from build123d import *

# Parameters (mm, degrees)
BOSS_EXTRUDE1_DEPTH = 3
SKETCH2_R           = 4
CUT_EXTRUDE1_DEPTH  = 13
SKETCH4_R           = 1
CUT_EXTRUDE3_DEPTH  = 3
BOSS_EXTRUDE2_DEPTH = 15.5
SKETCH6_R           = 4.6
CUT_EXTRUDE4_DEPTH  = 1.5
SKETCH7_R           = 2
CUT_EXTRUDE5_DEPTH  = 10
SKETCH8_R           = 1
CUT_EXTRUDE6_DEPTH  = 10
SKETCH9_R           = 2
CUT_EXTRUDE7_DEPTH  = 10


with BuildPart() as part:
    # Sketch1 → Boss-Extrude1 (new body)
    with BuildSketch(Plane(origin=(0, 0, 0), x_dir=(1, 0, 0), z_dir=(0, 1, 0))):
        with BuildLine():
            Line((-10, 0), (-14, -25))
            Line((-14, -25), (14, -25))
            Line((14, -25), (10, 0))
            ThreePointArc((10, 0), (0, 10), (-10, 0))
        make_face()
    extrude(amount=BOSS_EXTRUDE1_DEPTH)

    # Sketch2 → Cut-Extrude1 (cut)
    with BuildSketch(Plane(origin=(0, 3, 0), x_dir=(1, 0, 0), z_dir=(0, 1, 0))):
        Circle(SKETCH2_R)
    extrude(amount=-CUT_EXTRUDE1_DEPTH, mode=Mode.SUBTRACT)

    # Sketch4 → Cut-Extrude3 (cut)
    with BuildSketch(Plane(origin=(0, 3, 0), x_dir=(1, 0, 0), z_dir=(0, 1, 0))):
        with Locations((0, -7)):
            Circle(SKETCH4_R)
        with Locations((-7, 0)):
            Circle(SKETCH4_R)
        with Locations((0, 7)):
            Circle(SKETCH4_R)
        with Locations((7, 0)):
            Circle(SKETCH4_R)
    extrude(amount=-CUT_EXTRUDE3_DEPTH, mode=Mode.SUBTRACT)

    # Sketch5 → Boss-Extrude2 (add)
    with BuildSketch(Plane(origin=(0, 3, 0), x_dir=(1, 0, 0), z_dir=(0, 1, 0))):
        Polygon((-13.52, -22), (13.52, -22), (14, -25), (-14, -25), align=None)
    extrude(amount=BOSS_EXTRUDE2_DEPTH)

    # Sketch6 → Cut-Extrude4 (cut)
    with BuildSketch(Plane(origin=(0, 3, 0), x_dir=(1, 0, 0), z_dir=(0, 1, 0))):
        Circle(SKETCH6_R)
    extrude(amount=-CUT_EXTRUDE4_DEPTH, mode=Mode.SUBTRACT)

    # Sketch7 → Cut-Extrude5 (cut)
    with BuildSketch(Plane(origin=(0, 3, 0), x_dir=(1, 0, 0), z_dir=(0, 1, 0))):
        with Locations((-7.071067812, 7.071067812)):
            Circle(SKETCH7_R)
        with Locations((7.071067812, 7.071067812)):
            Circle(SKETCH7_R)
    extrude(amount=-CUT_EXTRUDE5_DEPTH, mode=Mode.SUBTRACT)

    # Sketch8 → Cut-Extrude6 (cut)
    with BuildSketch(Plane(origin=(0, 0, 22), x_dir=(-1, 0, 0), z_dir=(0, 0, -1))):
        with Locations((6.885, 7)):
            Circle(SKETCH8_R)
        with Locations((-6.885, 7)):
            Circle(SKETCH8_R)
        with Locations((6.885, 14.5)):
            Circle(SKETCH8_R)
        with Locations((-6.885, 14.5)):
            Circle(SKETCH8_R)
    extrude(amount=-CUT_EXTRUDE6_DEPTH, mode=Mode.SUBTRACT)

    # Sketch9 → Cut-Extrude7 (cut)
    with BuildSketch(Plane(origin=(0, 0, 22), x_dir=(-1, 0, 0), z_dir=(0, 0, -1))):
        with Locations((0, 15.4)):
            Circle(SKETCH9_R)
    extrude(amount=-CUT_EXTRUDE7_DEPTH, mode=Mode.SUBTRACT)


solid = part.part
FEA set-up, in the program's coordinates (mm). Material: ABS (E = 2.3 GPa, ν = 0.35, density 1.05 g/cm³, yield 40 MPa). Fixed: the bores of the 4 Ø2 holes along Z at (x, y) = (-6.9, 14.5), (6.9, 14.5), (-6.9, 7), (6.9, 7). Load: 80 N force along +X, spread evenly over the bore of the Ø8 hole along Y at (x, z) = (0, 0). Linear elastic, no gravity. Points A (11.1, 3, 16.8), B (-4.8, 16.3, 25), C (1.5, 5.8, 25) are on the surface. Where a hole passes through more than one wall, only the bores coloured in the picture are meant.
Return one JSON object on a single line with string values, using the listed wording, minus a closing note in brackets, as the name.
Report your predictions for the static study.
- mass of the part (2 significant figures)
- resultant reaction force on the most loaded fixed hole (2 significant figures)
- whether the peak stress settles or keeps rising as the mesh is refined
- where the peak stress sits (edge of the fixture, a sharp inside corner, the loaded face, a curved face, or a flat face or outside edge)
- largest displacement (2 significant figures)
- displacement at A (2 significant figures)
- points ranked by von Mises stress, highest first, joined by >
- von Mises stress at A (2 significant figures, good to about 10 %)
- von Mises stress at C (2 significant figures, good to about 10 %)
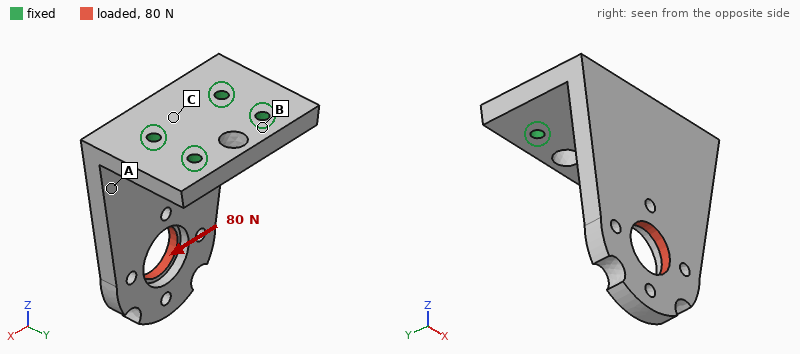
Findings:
{"mass of the part": "3.4 g", "resultant reaction force on the most loaded fixed hole": "130 N", "whether the peak stress settles or keeps rising as the mesh is refined": "keeps rising", "where the peak stress sits": "edge of the fixture", "largest displacement": "0.51 mm", "displacement at A": "0.18 mm", "points ranked by von Mises stress, highest first, joined by >": "A > C > B", "von Mises stress at A": "8.6 MPa", "von Mises stress at C": "4.9 MPa"}
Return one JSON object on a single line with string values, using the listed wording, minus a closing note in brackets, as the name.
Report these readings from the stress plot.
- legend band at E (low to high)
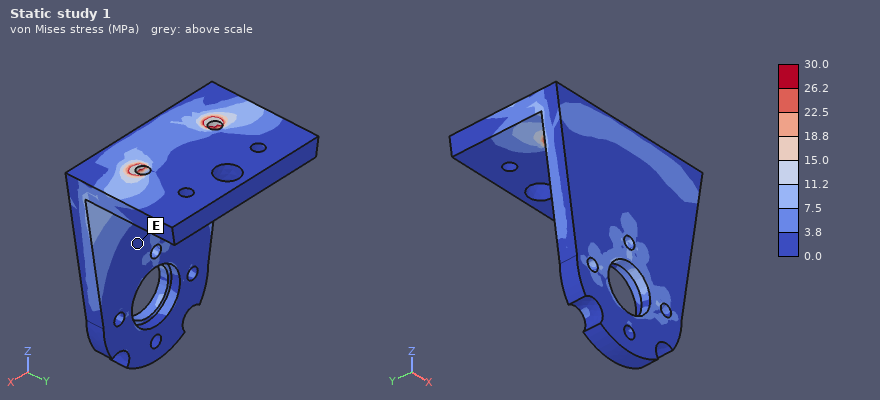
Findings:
{"legend band at E": "0.0 to 3.8 MPa"}
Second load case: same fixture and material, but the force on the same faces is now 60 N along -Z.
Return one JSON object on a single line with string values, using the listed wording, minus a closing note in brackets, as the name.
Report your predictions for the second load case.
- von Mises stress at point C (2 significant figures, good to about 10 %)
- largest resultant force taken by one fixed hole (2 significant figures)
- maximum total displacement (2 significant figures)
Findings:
{"von Mises stress at point C": "3.8 MPa", "largest resultant force taken by one fixed hole": "39 N", "maximum total displacement": "0.51 mm"}
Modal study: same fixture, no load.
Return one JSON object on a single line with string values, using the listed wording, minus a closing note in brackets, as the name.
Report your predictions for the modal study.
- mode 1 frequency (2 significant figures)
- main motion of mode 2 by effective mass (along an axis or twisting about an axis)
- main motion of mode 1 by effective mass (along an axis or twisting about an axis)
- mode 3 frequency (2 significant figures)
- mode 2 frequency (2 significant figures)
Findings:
{"mode 1 frequency": "740 Hz", "main motion of mode 2 by effective mass": "along X", "main motion of mode 1 by effective mass": "along Y", "mode 3 frequency": "2900 Hz", "mode 2 frequency": "2100 Hz"}
